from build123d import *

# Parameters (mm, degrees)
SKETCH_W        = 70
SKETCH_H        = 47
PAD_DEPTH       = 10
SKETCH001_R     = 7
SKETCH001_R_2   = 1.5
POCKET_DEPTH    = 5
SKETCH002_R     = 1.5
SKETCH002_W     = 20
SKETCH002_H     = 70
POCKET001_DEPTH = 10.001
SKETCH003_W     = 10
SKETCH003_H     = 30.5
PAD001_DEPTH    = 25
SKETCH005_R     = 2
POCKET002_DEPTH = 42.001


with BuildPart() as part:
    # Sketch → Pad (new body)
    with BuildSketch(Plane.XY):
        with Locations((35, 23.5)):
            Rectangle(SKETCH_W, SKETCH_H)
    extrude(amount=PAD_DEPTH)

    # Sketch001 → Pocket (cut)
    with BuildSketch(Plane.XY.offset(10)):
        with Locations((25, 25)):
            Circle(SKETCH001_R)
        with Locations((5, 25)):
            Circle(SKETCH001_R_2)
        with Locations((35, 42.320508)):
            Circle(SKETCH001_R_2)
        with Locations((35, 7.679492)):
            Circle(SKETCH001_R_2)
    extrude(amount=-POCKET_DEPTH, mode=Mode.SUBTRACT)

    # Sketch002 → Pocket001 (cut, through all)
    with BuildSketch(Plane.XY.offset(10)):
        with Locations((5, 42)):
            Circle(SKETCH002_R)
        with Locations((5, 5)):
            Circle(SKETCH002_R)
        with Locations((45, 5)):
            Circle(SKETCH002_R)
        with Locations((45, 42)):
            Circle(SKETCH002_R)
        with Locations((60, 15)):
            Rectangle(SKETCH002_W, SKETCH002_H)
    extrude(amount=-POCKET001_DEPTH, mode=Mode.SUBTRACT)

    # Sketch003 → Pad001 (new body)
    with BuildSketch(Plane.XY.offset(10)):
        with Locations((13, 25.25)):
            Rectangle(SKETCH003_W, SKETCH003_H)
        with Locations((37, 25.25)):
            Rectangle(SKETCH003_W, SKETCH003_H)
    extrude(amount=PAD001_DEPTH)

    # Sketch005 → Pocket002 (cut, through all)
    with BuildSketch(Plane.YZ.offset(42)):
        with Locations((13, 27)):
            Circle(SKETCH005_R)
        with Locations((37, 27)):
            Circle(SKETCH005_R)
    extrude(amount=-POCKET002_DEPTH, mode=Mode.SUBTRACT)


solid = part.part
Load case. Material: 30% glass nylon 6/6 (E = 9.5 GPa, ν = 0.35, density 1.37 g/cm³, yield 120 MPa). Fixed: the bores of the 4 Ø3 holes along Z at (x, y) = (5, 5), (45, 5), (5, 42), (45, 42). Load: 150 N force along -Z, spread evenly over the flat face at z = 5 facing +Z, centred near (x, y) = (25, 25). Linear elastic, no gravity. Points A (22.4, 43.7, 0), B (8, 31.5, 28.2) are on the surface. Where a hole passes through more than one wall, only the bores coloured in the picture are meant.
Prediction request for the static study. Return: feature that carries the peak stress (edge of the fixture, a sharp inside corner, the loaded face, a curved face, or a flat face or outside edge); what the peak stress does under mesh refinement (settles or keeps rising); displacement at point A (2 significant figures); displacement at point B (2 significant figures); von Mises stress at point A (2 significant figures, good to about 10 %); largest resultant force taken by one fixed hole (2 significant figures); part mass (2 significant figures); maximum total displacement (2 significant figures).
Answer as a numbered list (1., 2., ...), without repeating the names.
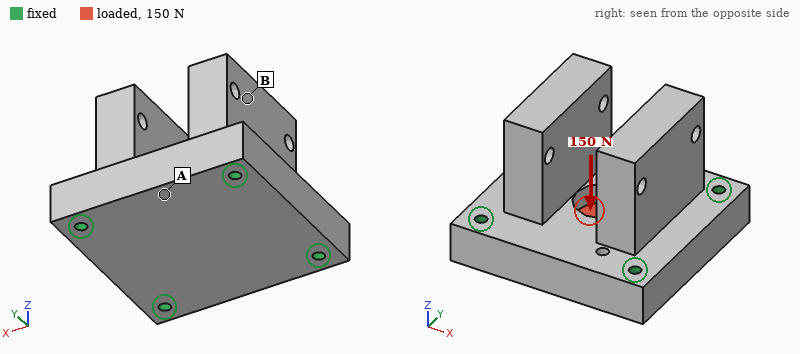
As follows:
1. edge of the fixture
2. keeps rising
3. 2.6 µm
4. 4.8 µm
5. 0.74 MPa
6. 41 N
7. 51 g
8. 6.9 µm
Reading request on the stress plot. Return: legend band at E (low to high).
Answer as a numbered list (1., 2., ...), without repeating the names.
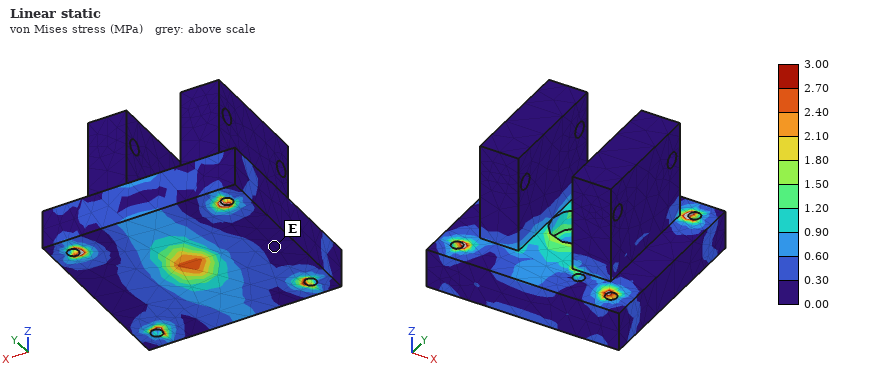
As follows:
1. 0.00 to 0.30 MPa
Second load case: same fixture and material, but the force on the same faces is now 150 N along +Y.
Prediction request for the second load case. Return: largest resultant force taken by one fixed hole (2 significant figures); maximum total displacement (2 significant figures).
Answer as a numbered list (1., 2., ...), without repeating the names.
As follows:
1. 43 N
2. 2.2 µm
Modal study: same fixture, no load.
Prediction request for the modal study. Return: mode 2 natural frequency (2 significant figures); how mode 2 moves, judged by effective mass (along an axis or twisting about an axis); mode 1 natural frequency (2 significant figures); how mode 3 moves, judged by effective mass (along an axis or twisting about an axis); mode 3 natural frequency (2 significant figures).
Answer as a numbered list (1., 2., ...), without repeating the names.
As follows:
1. 4600 Hz
2. along X
3. 3800 Hz
4. along Y
5. 7000 Hz
